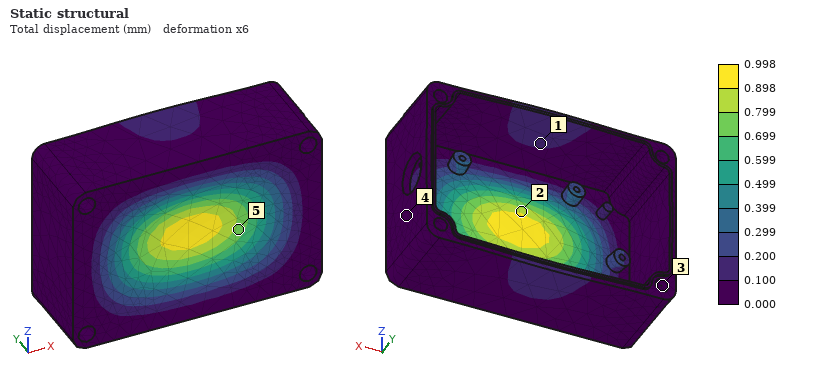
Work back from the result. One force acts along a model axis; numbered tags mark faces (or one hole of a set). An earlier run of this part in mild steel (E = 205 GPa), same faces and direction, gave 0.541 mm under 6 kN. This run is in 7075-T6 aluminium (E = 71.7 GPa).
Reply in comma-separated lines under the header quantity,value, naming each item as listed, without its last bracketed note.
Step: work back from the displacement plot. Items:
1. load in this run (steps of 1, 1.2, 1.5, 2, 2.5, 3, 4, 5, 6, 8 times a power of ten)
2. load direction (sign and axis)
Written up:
quantity,value
load in this run,4 kN
load direction,+Y
